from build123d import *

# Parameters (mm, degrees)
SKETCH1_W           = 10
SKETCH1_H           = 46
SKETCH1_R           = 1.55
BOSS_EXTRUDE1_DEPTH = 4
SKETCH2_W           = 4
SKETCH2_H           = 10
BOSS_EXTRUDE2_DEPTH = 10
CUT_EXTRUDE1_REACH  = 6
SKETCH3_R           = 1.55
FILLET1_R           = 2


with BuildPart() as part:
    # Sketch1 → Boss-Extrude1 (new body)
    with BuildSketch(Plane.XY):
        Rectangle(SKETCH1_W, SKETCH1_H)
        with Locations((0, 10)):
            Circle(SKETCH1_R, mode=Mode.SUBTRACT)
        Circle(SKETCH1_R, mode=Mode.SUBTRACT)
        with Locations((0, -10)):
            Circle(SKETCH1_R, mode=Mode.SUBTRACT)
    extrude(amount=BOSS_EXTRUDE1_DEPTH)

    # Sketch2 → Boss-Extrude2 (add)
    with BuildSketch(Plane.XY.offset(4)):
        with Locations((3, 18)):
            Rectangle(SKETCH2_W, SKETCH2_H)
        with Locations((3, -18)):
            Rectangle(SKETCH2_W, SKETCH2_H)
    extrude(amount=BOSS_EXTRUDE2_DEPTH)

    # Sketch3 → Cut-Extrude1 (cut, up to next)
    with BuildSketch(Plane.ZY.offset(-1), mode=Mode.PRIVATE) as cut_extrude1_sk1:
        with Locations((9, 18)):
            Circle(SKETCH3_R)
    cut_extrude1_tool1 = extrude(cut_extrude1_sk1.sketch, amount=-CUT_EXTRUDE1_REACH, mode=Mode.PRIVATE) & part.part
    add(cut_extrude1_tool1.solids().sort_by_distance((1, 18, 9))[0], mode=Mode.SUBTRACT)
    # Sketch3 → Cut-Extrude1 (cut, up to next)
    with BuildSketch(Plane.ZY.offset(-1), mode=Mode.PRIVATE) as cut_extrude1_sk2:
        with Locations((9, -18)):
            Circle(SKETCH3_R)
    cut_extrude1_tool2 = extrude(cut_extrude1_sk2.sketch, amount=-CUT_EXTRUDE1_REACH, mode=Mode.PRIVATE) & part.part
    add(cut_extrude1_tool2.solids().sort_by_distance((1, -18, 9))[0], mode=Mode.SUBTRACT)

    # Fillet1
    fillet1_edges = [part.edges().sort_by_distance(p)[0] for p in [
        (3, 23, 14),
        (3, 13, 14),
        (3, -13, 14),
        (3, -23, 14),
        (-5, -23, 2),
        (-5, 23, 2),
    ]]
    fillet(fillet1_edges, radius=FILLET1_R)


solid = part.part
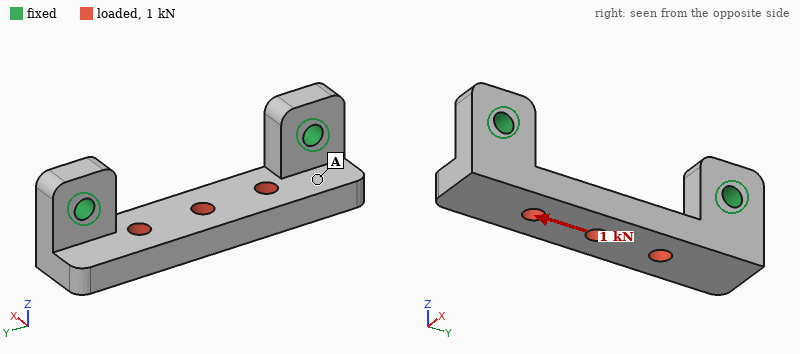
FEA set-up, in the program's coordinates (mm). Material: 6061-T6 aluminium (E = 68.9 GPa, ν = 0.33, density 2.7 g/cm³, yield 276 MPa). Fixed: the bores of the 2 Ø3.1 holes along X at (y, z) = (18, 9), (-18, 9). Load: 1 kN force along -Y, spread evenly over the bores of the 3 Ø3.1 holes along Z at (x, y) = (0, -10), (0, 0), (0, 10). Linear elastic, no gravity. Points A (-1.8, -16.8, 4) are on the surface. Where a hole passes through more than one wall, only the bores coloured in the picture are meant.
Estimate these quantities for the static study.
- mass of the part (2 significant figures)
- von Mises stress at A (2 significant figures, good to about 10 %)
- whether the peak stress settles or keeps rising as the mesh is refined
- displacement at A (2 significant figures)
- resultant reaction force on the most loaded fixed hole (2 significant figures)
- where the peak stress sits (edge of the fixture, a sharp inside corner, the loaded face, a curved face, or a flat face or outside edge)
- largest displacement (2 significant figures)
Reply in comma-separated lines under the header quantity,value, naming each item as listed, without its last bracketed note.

quantity,value
mass of the part,6.7 g
von Mises stress at A,14 MPa
whether the peak stress settles or keeps rising as the mesh is refined,keeps rising
displacement at A,8.9 µm
resultant reaction force on the most loaded fixed hole,510 N
where the peak stress sits,edge of the fixture
largest displacement,13 µm
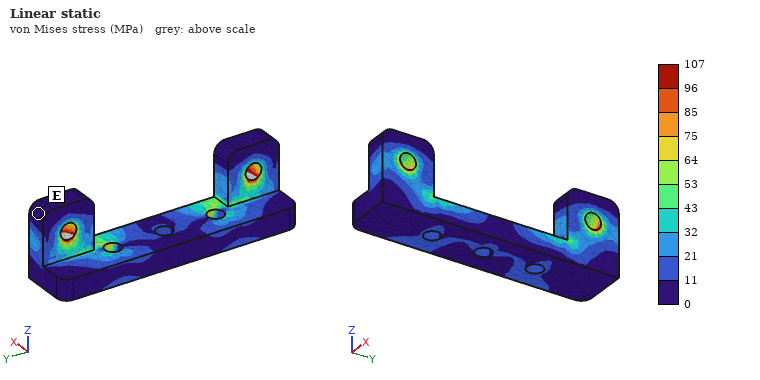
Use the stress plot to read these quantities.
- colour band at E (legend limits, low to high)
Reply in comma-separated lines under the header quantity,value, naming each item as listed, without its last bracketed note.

quantity,value
colour band at E,0 to 11 MPa
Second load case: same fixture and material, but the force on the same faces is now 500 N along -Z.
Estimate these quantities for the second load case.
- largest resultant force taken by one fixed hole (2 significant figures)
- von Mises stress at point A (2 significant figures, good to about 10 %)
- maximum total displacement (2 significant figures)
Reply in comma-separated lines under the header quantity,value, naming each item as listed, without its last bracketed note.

quantity,value
largest resultant force taken by one fixed hole,300 N
von Mises stress at point A,21 MPa
maximum total displacement,37 µm
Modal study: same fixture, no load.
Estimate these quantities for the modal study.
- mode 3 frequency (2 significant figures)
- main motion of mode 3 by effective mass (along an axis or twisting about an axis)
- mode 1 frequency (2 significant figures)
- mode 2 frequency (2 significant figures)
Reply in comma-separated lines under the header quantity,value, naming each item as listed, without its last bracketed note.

quantity,value
mode 3 frequency,19 kHz
main motion of mode 3 by effective mass,along Y
mode 1 frequency,11 kHz
mode 2 frequency,18 kHz
